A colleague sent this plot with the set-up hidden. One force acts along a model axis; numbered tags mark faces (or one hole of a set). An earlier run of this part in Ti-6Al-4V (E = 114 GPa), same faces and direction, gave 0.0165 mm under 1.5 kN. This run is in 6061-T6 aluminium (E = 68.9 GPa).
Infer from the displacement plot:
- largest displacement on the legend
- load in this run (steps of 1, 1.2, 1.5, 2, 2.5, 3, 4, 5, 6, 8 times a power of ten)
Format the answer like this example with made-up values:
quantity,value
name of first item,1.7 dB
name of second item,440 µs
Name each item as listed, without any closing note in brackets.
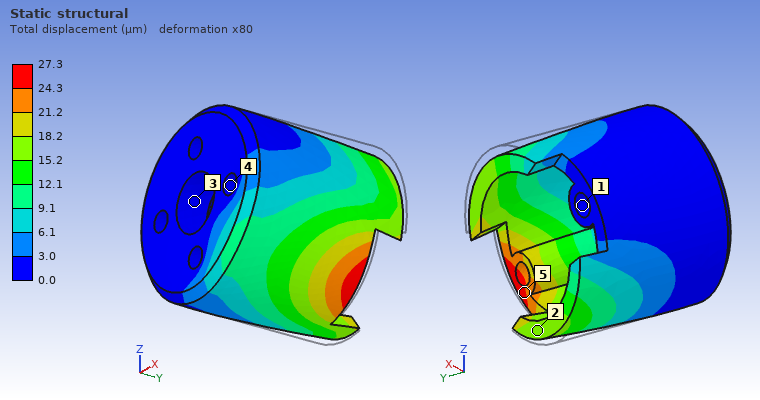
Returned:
quantity,value
largest displacement on the legend,27.3 µm
load in this run,1.5 kN
